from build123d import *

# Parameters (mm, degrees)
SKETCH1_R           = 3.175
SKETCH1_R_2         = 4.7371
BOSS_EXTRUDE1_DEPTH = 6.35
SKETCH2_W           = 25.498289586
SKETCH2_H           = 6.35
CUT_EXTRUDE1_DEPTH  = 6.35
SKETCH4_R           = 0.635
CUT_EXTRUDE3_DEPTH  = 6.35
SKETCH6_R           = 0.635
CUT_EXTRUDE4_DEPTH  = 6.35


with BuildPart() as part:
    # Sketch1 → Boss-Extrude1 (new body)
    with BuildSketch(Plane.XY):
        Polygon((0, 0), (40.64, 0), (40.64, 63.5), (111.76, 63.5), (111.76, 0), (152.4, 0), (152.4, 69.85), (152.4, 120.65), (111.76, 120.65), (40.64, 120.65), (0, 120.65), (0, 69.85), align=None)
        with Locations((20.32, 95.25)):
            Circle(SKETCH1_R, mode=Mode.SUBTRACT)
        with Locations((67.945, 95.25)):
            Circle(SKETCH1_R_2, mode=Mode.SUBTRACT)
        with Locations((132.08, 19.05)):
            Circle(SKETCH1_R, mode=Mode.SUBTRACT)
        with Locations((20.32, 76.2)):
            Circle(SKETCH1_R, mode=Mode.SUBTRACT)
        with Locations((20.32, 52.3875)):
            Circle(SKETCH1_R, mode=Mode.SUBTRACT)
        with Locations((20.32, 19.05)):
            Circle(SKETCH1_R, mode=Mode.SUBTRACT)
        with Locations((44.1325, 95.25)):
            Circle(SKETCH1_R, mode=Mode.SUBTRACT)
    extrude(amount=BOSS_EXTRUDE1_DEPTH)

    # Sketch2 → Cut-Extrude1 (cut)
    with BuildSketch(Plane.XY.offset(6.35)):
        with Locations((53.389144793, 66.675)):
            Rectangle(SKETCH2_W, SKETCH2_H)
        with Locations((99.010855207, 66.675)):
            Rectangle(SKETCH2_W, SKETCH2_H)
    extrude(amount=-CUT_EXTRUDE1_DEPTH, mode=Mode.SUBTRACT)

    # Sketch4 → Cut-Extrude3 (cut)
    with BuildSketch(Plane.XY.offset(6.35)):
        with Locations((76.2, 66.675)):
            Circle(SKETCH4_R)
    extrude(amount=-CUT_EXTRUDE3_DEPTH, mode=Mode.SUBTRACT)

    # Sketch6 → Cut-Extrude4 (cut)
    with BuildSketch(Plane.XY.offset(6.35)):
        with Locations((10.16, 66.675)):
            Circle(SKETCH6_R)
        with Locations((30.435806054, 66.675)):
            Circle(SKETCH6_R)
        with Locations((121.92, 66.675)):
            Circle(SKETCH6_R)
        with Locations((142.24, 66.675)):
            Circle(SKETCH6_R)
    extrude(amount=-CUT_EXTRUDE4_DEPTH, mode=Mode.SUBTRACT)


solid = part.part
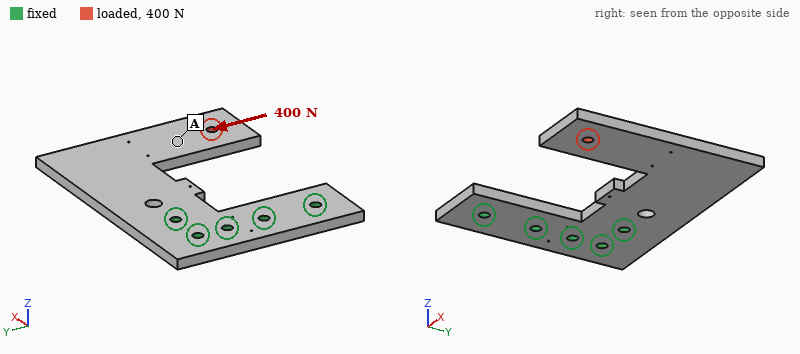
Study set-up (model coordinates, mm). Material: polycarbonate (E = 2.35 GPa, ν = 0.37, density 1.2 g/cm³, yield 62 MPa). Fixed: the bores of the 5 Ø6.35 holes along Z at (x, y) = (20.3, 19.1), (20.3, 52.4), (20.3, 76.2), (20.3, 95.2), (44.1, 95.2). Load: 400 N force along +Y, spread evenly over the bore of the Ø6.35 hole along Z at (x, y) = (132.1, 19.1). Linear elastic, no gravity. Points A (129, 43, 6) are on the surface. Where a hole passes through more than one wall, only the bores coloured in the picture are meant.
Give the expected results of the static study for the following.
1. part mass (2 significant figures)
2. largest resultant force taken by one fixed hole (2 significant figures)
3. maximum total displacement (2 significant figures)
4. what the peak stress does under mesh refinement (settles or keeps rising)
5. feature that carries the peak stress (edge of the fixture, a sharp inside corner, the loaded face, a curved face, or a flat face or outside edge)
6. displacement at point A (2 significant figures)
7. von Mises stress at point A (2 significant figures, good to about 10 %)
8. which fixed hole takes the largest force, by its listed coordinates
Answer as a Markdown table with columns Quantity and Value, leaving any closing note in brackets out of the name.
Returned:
| Quantity | Value |
|---|---|
| part mass | 100 g |
| largest resultant force taken by one fixed hole | 930 N |
| maximum total displacement | 2.0 mm |
| what the peak stress does under mesh refinement | keeps rising |
| feature that carries the peak stress | edge of the fixture |
| displacement at point A | 1.3 mm |
| von Mises stress at point A | 1.7 MPa |
| which fixed hole takes the largest force, by its listed coordinates | (44.1, 95.2) |
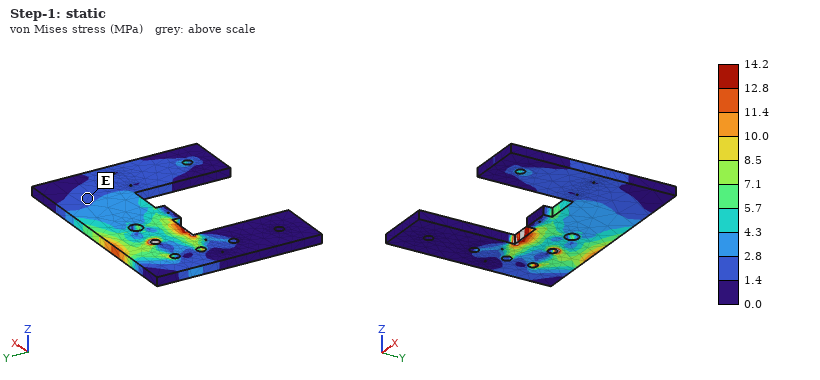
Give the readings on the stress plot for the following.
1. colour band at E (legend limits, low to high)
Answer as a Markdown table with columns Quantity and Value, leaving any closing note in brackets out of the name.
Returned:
| Quantity | Value |
|---|---|
| colour band at E | 1.4 to 2.8 MPa |
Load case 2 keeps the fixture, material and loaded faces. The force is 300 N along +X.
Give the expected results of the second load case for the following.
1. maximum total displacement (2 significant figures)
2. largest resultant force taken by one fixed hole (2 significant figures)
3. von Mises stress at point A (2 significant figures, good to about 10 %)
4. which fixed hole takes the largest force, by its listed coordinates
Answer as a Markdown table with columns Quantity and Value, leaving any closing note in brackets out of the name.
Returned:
| Quantity | Value |
|---|---|
| maximum total displacement | 2.3 mm |
| largest resultant force taken by one fixed hole | 420 N |
| von Mises stress at point A | 3.0 MPa |
| which fixed hole takes the largest force, by its listed coordinates | (20.3, 76.2) |
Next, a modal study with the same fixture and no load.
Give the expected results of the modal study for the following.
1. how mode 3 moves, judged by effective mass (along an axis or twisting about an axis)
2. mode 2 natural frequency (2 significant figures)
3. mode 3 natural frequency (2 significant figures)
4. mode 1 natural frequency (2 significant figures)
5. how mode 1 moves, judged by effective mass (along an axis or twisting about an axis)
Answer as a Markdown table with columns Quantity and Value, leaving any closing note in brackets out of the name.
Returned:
| Quantity | Value |
|---|---|
| how mode 3 moves, judged by effective mass | along Y |
| mode 2 natural frequency | 160 Hz |
| mode 3 natural frequency | 390 Hz |
| mode 1 natural frequency | 69 Hz |
| how mode 1 moves, judged by effective mass | along Z |
